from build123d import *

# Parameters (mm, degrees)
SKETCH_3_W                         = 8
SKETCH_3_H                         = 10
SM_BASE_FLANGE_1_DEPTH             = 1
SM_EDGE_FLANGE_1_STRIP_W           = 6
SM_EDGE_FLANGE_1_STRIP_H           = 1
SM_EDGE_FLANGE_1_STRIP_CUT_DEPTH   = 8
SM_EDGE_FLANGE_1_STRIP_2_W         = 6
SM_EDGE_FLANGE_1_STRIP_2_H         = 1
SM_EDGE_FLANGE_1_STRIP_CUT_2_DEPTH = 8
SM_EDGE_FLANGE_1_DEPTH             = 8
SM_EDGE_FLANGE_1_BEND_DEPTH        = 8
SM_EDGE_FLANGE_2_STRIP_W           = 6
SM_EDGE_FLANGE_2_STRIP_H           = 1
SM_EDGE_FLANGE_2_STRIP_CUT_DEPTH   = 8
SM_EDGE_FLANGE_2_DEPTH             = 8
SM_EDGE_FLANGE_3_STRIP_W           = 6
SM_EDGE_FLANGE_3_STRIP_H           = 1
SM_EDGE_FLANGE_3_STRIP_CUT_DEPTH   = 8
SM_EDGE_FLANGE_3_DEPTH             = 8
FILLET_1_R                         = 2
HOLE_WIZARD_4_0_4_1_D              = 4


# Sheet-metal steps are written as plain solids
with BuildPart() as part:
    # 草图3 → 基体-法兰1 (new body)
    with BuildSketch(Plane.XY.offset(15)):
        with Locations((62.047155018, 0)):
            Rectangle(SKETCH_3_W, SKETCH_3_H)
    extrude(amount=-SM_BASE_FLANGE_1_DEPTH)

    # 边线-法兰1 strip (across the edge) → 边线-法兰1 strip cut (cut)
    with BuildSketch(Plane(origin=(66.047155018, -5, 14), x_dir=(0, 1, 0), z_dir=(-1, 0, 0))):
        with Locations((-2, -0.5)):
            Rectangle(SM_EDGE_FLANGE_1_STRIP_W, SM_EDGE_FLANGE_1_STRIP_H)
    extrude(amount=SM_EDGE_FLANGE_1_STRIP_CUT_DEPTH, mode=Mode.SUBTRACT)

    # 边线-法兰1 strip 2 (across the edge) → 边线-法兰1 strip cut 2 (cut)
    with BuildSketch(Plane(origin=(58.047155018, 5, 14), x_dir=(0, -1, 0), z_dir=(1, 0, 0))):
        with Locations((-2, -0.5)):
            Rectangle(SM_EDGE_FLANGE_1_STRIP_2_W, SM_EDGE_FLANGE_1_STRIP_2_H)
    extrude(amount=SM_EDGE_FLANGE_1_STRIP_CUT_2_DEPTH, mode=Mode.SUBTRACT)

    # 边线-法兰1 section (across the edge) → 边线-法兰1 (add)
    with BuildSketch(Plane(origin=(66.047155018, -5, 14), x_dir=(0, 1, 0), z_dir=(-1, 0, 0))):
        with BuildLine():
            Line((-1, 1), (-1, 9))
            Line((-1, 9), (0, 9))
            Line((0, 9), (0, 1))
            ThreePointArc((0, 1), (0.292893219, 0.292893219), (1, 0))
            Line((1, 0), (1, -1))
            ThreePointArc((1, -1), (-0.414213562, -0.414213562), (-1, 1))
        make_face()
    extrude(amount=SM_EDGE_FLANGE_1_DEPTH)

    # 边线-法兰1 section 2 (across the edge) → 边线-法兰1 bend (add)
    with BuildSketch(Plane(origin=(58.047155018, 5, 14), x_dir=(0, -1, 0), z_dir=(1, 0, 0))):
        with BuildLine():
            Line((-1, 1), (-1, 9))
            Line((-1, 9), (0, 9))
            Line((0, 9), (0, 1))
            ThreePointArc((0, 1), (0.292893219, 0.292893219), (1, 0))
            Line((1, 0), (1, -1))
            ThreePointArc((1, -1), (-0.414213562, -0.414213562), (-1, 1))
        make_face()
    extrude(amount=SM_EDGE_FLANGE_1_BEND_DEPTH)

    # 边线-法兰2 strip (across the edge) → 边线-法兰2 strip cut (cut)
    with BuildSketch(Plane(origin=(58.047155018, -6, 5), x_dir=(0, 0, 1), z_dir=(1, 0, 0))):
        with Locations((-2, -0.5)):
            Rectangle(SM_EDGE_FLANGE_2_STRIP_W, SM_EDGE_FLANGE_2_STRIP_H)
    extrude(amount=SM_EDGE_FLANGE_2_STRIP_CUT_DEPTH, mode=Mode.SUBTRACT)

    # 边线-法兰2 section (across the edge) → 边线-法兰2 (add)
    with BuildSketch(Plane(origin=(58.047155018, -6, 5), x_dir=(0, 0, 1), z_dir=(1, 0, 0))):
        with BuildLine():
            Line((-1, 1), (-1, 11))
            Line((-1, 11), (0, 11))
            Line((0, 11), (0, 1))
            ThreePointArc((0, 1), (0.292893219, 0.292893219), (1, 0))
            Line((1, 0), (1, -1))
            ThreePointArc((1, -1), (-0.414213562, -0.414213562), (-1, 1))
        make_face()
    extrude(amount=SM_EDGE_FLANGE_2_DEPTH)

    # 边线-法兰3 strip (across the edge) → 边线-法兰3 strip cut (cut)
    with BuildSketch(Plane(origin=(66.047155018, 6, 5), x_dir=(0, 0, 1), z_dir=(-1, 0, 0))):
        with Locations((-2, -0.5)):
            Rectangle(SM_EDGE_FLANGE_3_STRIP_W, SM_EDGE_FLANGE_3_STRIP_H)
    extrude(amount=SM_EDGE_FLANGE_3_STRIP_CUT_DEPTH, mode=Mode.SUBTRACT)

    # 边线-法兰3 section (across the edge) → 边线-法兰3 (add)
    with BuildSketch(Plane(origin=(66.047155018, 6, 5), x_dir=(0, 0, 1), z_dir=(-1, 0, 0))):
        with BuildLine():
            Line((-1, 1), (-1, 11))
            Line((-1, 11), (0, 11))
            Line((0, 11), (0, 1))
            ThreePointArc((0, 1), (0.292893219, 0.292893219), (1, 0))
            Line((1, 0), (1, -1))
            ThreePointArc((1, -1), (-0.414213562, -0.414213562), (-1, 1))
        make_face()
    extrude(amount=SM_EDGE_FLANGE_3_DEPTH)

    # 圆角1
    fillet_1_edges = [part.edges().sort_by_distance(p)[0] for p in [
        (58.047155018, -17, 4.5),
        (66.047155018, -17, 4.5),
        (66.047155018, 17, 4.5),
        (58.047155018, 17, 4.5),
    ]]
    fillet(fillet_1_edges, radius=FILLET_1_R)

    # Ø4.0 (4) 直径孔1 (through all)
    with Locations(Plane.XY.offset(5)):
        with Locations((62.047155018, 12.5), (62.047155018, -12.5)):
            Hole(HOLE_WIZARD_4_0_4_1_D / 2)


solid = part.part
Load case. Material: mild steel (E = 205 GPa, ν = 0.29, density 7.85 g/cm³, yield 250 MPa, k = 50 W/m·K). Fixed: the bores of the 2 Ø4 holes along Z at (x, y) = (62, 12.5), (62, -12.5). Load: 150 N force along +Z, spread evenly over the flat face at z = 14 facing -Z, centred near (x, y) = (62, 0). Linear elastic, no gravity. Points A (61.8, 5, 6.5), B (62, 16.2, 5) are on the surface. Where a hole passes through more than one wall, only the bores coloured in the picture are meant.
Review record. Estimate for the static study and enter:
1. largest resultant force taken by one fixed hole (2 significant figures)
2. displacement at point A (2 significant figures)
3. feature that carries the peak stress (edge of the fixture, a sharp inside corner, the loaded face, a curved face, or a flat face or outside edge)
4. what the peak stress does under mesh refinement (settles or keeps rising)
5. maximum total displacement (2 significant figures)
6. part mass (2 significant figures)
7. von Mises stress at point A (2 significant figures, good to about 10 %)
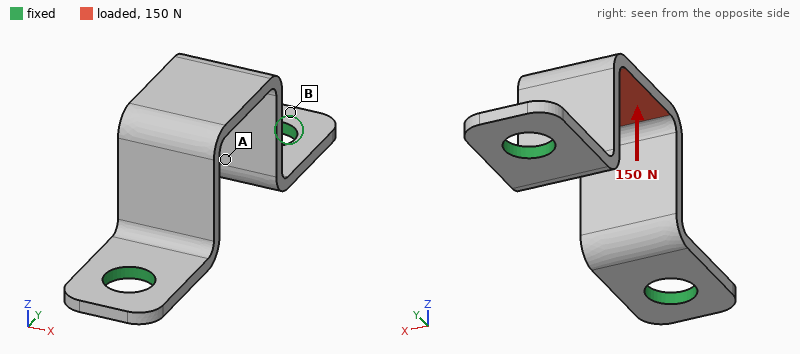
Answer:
82 N
12 µm
edge of the fixture
keeps rising
20 µm
3.0 g
60 MPa
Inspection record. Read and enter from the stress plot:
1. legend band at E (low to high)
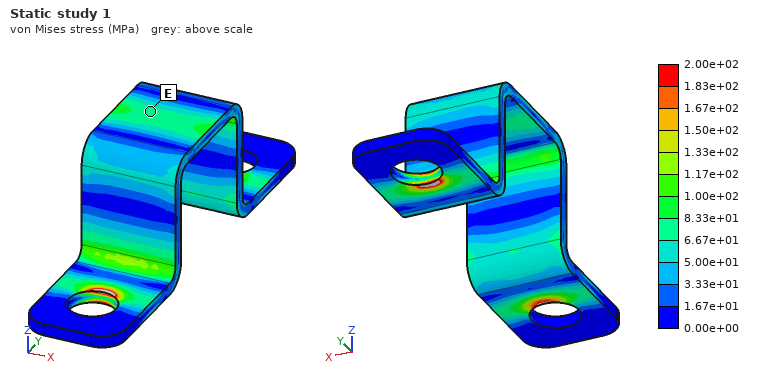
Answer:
6.67e+01 to 8.33e+01 MPa
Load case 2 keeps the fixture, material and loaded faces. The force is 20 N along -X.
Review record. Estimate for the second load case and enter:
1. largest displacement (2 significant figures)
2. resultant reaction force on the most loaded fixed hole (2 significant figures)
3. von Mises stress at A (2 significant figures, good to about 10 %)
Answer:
19 µm
10 N
6.0 MPa
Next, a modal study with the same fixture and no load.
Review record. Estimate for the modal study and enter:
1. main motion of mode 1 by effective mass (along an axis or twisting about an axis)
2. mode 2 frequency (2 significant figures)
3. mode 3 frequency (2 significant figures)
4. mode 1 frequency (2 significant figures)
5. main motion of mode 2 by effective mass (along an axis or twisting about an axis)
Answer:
along X
6800 Hz
10 kHz
5000 Hz
along Y
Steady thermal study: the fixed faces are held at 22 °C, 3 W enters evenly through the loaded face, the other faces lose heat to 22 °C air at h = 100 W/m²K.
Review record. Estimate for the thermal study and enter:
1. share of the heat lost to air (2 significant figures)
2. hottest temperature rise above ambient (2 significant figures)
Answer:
46 %
46 K
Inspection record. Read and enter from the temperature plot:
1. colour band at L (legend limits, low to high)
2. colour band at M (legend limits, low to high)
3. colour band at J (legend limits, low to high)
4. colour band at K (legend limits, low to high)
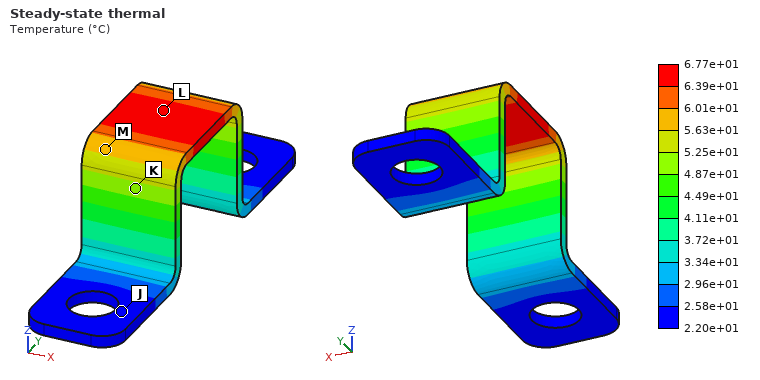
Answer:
6.39e+01 to 6.77e+01 °C
5.63e+01 to 6.01e+01 °C
2.20e+01 to 2.58e+01 °C
4.87e+01 to 5.25e+01 °C
